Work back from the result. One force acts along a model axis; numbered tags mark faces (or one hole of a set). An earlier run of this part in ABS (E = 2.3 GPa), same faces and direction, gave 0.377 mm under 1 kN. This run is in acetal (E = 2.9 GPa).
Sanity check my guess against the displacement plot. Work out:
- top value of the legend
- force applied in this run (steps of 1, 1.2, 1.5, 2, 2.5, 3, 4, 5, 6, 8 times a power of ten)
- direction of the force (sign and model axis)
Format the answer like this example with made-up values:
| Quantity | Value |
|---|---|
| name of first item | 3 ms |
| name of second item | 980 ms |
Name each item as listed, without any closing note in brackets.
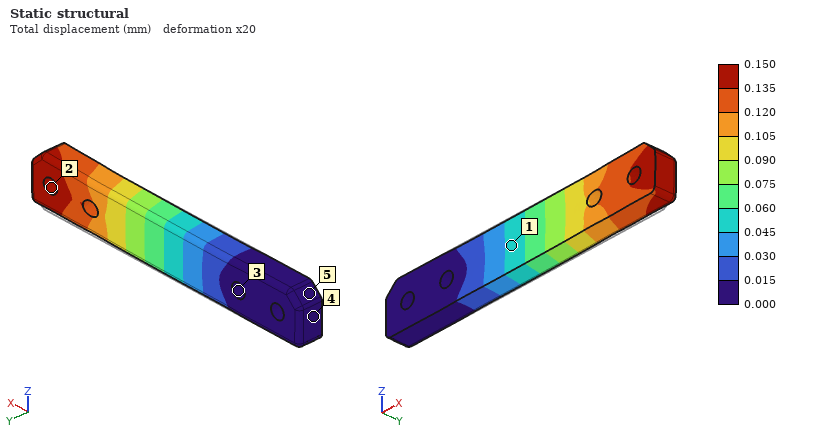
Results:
| Quantity | Value |
|---|---|
| top value of the legend | 0.150 mm |
| force applied in this run | 500 N |
| direction of the force | +X |
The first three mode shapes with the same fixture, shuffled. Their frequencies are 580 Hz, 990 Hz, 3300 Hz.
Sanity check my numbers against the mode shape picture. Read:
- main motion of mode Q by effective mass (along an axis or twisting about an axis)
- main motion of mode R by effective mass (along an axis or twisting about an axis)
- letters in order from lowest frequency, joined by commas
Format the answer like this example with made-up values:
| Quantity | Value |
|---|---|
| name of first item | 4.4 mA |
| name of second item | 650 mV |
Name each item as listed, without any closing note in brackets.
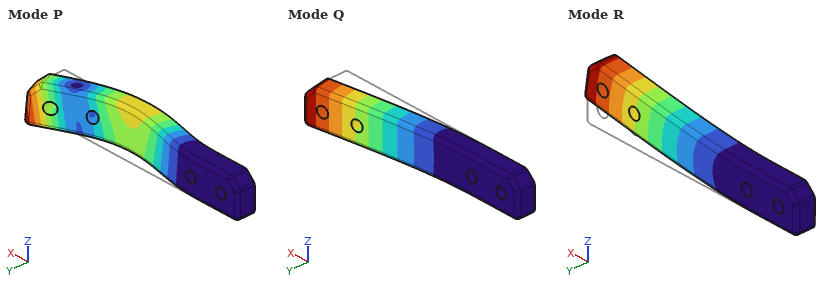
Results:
| Quantity | Value |
|---|---|
| main motion of mode Q by effective mass | along Y |
| main motion of mode R by effective mass | along Z |
| letters in order from lowest frequency, joined by commas | Q, R, P |
